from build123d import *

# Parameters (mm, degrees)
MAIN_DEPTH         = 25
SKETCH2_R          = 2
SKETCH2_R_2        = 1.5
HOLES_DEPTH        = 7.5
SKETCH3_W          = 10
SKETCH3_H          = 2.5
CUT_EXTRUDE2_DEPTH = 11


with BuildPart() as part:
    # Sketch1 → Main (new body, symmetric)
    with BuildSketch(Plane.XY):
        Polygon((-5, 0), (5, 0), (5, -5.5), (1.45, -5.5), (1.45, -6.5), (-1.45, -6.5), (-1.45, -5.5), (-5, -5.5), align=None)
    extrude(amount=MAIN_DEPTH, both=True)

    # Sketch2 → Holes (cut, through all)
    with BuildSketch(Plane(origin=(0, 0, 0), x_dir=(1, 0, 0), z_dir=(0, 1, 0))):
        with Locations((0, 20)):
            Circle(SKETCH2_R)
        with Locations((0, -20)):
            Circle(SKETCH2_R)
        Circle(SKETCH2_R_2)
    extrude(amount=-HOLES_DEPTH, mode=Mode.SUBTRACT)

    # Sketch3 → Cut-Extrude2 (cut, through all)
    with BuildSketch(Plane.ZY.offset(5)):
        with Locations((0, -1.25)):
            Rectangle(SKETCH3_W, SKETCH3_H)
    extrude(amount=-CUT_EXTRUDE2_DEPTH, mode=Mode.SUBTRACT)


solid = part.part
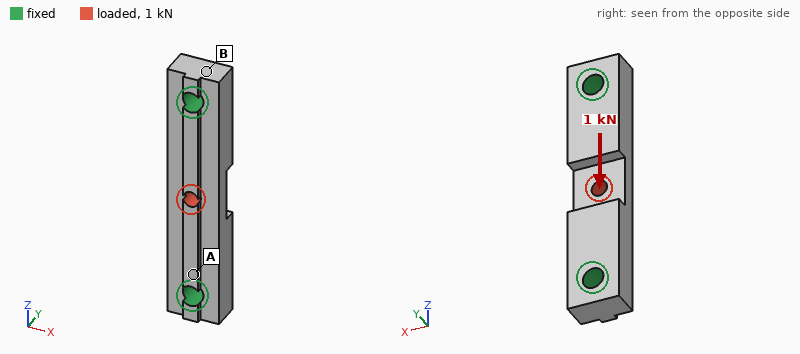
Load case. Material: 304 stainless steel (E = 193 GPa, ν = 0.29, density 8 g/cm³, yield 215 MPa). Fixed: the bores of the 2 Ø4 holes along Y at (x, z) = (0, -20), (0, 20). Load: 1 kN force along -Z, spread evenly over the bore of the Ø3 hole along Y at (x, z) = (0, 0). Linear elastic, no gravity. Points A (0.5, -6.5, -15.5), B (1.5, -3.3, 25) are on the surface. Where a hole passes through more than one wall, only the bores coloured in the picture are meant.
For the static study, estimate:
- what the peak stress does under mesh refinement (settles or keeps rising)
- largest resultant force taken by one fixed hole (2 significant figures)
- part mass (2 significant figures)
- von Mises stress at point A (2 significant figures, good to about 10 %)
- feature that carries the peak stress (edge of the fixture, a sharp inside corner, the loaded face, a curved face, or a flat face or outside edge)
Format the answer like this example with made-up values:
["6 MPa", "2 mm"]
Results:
["keeps rising", "500 N", "20 g", "11 MPa", "a sharp inside corner"]
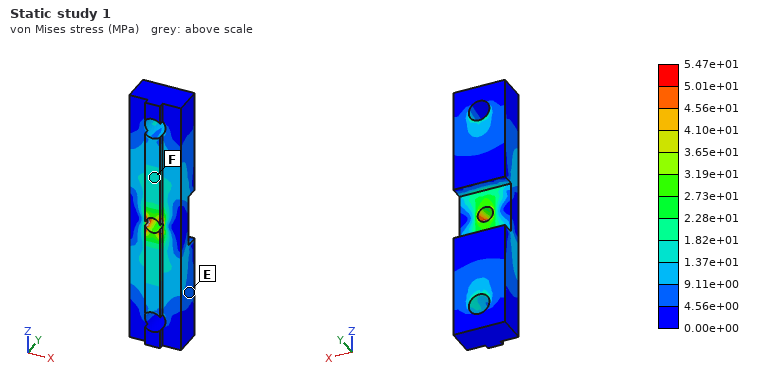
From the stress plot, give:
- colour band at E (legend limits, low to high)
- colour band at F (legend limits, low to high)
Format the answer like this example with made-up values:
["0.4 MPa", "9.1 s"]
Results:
["4.56e+00 to 9.11e+00 MPa", "1.37e+01 to 1.82e+01 MPa"]
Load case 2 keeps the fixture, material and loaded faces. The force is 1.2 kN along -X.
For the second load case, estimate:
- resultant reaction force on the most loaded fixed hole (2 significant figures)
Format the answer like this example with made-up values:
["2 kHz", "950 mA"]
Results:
["600 N"]
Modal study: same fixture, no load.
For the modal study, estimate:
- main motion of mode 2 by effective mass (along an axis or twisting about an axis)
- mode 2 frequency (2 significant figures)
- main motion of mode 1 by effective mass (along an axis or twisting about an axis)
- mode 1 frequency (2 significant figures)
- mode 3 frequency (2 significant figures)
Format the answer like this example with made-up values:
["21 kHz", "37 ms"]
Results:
["along X", "23 kHz", "along Y", "18 kHz", "35 kHz"]
